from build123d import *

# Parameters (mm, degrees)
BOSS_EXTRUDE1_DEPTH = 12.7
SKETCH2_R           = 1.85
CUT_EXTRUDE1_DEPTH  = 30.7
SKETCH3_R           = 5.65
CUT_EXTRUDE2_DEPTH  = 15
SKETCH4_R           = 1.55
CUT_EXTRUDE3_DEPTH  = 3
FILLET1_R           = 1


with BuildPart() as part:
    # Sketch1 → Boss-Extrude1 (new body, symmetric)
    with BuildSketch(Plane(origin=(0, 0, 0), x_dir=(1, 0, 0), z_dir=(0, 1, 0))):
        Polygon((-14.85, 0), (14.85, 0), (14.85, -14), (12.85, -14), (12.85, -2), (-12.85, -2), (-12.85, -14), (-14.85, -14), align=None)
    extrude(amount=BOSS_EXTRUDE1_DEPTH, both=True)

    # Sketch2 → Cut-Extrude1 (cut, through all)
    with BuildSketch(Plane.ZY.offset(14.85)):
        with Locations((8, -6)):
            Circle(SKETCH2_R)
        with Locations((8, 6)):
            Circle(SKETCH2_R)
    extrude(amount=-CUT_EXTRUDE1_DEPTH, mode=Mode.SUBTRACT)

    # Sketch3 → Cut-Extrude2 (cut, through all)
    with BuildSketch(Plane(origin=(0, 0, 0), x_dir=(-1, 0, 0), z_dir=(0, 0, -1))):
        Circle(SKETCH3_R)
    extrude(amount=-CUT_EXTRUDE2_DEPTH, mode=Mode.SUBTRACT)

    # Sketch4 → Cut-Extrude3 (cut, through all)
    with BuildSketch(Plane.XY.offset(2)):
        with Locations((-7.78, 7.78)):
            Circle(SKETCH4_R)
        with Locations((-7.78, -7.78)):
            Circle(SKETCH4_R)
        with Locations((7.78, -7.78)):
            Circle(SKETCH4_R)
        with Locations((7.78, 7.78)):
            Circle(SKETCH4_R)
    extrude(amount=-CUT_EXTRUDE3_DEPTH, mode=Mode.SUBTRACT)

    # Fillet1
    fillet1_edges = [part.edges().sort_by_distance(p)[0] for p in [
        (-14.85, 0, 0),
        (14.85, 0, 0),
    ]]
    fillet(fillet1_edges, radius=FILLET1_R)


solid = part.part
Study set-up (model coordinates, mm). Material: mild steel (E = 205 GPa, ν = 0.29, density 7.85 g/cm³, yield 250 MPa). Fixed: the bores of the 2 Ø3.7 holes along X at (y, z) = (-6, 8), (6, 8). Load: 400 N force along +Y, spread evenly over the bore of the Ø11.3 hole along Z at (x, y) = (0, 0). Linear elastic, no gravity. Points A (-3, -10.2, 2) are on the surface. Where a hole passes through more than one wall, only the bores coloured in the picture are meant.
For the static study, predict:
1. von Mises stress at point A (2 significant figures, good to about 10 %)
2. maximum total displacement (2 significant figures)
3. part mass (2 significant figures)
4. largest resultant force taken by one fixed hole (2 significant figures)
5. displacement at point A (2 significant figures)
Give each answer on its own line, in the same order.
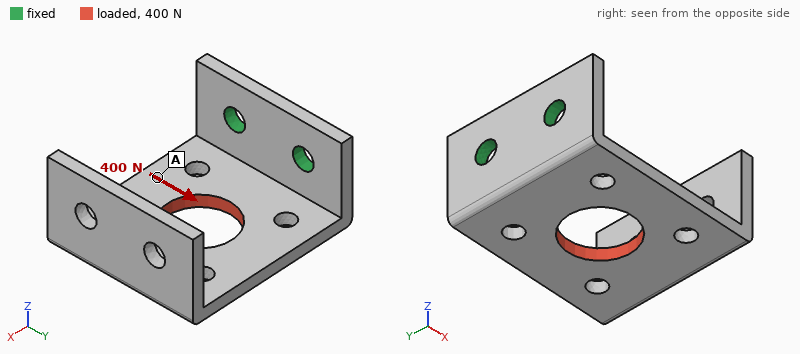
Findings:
38 MPa
78 µm
19 g
440 N
30 µm
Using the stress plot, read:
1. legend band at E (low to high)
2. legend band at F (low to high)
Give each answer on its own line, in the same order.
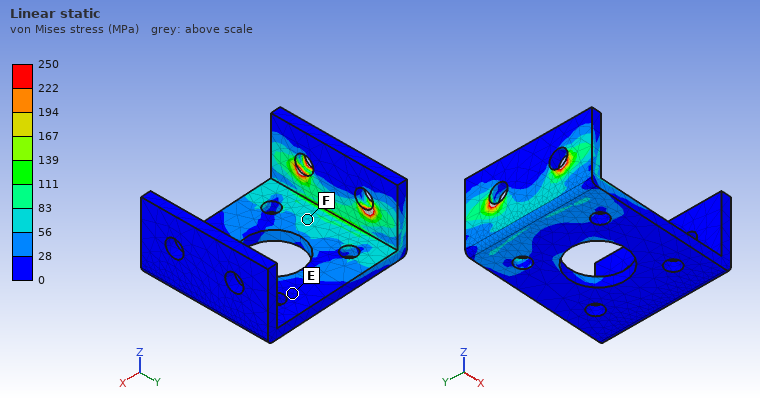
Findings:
0 to 28 MPa
56 to 83 MPa
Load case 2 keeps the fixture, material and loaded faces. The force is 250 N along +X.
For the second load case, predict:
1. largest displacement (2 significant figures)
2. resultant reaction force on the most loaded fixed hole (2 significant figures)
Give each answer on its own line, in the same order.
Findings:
40 µm
130 N
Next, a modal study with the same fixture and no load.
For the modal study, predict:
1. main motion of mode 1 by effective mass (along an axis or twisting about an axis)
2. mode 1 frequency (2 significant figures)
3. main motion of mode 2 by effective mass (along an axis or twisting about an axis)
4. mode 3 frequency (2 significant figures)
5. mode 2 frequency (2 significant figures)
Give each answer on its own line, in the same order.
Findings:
along Z
900 Hz
along Y
4100 Hz
2100 Hz
